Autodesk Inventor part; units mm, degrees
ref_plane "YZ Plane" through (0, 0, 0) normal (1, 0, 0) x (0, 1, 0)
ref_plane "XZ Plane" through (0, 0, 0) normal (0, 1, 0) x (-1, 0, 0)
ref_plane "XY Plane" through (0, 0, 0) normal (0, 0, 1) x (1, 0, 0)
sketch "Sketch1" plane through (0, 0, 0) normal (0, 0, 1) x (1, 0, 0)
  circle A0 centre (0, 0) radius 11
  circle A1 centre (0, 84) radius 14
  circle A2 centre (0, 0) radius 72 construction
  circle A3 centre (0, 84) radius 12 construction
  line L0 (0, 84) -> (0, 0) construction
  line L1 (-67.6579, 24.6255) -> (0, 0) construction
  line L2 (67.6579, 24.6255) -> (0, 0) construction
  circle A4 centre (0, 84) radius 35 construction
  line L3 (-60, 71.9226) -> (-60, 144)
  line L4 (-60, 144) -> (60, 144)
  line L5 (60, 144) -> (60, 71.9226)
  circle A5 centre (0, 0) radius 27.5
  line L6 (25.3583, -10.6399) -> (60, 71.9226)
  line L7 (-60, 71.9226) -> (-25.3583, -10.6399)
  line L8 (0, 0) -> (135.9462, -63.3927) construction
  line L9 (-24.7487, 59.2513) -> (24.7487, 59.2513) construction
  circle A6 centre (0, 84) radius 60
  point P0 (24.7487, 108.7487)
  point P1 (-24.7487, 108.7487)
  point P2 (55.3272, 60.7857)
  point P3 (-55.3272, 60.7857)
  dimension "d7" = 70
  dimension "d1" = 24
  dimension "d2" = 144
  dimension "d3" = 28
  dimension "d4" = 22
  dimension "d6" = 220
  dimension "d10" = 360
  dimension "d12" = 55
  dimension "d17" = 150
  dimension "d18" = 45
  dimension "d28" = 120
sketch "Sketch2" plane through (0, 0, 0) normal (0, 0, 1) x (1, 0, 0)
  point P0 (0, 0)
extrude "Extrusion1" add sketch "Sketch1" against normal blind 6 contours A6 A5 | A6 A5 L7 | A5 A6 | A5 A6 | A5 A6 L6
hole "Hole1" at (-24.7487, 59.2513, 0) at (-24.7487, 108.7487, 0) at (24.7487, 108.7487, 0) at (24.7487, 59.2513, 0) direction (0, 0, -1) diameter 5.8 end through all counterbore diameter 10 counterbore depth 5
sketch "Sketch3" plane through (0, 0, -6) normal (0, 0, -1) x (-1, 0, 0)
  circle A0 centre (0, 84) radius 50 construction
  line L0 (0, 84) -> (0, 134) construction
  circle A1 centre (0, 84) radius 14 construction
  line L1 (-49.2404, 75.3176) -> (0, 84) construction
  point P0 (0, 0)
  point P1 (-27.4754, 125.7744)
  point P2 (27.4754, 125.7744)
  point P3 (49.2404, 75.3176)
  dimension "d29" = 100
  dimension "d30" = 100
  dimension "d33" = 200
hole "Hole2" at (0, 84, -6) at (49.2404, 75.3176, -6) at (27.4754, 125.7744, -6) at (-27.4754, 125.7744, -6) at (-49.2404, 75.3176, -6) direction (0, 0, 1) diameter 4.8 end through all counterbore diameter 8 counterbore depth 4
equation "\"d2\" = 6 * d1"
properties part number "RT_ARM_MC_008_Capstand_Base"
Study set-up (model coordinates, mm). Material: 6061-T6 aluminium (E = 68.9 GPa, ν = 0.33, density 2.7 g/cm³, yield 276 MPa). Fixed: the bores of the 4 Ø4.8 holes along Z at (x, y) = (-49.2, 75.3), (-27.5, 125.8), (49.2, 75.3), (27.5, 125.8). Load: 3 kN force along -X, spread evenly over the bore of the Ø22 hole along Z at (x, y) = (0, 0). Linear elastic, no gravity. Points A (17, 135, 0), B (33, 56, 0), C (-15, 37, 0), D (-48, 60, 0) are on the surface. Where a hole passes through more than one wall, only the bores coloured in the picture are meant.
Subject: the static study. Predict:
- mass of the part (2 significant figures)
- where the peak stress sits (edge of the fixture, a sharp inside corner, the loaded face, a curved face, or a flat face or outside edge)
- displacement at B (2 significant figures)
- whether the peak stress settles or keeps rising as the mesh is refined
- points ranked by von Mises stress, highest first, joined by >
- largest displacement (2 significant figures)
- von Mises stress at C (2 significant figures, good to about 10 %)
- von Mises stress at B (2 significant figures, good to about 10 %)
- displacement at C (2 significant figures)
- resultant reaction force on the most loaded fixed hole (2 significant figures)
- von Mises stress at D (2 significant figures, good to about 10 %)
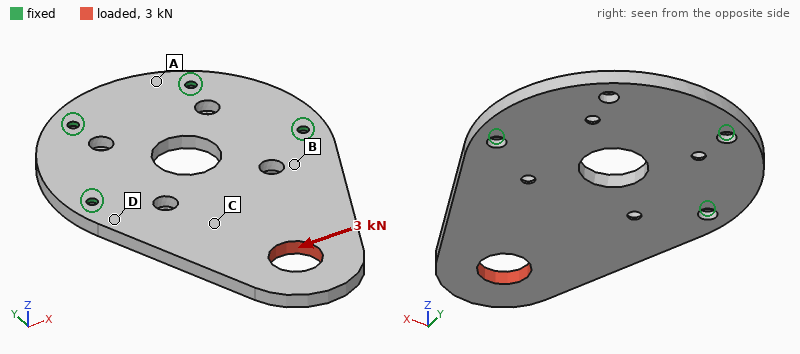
220 g
edge of the fixture
19 µm
keeps rising
D > B > C > A
59 µm
11 MPa
21 MPa
23 µm
2.5 kN
27 MPa
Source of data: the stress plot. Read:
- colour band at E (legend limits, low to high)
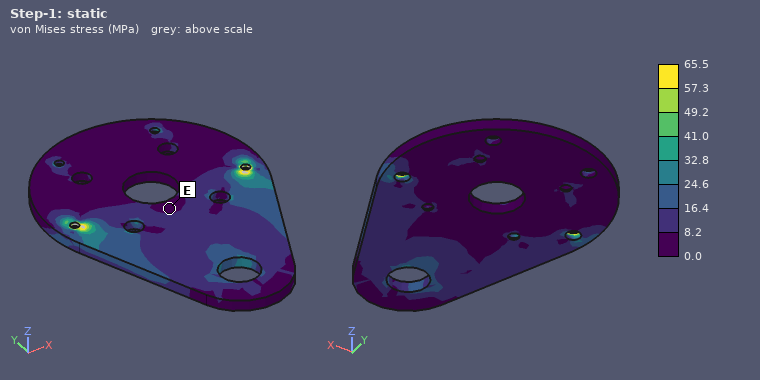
0.0 to 8.2 MPa
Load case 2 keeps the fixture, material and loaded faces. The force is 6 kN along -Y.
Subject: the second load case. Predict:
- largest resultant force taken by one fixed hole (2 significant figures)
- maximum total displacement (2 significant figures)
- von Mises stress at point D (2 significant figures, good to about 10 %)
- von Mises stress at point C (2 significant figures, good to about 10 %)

2.0 kN
0.11 mm
17 MPa
11 MPa
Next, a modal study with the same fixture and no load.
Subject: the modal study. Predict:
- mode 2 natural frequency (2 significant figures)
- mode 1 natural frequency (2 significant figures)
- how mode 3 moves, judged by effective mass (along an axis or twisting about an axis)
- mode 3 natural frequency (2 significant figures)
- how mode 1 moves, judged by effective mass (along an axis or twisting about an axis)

2000 Hz
500 Hz
along Z
2200 Hz
along Z
